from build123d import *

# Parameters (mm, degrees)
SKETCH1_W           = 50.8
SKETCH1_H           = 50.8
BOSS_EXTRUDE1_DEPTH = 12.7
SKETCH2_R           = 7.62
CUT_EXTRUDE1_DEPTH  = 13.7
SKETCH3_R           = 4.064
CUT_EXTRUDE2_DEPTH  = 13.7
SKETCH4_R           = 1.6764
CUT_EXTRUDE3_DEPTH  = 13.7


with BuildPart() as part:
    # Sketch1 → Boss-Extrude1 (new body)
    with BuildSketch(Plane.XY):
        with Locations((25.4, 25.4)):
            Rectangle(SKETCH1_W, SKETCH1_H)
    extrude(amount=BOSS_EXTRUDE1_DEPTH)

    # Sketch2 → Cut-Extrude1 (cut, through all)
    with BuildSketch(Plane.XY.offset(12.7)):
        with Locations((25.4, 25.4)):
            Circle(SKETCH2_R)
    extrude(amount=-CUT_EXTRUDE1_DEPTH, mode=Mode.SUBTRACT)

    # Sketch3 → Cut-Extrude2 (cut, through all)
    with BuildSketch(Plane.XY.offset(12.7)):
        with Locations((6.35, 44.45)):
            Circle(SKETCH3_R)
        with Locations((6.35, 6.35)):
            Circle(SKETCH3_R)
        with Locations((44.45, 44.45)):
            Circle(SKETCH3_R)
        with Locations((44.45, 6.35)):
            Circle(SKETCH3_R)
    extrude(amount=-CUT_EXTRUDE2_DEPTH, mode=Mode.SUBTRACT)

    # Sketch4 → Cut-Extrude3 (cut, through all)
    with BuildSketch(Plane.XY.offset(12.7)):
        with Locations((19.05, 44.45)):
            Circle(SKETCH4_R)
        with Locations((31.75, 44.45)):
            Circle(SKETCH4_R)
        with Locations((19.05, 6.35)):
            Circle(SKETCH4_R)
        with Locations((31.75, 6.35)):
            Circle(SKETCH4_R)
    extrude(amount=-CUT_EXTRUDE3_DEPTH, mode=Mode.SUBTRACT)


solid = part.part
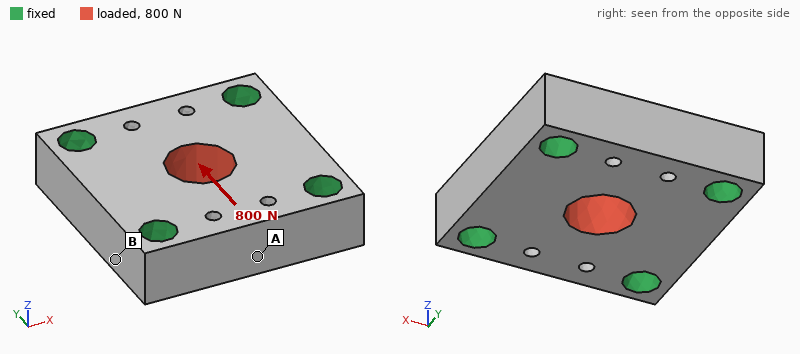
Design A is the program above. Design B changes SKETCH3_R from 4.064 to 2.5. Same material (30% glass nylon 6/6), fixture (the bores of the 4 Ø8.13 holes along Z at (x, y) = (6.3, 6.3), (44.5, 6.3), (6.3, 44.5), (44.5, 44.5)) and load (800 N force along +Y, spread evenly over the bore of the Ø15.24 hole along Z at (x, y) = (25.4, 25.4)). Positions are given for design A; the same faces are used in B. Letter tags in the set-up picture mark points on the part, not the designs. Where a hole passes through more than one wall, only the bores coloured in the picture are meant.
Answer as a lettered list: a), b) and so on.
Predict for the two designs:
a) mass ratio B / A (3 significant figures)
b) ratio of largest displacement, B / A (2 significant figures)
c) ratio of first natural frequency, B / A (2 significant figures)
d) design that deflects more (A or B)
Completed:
a) 1.06
b) 1.1
c) 0.84
d) B
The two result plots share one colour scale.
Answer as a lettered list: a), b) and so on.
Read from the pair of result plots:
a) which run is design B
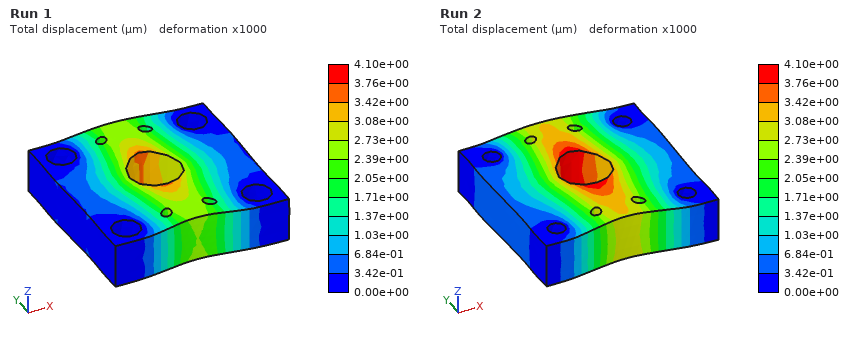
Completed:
a) Run 2
